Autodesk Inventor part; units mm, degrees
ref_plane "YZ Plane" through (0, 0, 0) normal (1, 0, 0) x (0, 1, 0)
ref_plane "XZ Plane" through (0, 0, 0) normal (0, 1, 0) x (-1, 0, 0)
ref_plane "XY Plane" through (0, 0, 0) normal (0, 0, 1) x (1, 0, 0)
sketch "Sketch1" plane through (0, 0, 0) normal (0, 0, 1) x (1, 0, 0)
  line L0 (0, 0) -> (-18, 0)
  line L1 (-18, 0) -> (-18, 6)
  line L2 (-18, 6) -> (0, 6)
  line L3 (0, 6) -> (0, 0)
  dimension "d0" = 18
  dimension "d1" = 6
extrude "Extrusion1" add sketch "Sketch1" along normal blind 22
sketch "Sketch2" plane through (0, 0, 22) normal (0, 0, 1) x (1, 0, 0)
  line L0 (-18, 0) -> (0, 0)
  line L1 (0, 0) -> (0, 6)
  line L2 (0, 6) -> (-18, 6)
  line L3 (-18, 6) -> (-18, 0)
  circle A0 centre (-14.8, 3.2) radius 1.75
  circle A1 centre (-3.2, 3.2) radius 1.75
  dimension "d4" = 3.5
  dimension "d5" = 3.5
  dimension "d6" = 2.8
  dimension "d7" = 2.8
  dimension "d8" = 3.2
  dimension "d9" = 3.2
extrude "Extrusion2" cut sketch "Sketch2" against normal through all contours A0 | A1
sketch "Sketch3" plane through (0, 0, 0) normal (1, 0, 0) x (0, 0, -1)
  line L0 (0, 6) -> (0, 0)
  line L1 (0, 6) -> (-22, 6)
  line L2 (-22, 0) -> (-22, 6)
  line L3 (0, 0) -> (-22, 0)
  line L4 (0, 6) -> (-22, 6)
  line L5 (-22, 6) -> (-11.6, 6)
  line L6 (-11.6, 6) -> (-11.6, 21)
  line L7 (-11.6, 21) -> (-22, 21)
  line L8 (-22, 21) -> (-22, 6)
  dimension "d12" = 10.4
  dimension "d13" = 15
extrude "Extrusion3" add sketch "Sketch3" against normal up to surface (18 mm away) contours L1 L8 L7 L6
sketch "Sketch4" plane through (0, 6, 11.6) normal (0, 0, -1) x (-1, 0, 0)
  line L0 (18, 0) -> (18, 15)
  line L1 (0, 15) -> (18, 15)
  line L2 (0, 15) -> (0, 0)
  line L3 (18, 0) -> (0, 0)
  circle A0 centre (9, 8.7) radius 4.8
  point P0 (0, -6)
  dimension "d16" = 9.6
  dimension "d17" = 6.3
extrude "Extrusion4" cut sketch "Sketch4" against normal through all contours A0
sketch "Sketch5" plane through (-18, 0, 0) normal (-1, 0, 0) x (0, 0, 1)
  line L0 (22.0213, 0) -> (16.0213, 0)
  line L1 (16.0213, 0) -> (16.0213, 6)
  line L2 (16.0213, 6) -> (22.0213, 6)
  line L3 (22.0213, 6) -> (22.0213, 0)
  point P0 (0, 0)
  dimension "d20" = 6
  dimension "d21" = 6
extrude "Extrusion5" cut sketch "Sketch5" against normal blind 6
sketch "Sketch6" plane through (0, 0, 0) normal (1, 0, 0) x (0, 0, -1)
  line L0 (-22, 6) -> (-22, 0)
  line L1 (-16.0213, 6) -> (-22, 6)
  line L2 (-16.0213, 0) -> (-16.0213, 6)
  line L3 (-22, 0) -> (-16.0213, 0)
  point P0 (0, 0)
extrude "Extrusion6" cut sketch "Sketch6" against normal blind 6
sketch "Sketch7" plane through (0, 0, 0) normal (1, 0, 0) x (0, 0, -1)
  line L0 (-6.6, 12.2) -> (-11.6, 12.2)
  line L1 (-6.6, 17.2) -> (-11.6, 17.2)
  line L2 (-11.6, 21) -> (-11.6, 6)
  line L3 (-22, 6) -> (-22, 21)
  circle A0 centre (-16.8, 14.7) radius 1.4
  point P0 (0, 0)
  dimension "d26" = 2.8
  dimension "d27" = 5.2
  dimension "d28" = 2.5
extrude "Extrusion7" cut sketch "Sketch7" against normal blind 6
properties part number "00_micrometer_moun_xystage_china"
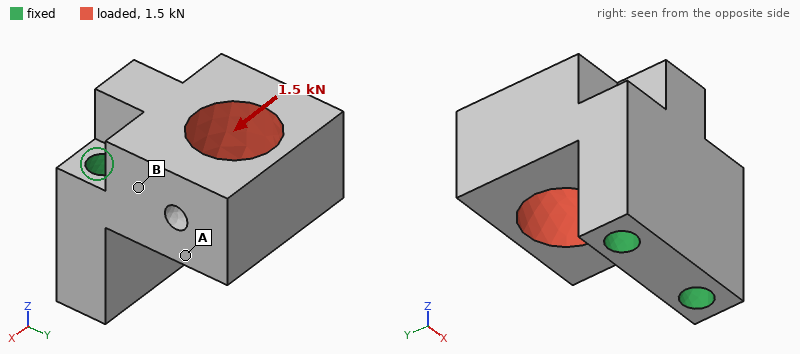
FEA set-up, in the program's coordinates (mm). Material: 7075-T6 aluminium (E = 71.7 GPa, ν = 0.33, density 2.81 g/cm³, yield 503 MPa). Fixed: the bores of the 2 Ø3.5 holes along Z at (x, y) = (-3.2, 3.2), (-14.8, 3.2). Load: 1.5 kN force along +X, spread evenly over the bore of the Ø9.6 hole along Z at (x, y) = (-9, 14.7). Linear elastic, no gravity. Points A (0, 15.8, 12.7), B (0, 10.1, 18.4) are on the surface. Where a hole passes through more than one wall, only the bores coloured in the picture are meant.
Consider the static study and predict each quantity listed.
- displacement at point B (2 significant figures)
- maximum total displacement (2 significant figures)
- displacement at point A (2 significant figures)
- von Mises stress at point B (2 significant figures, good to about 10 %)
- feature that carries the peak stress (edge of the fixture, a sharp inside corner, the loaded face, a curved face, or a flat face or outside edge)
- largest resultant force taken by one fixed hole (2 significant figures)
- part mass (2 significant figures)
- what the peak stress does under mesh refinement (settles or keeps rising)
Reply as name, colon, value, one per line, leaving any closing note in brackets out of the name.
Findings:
displacement at point B: 10 µm
maximum total displacement: 30 µm
displacement at point A: 20 µm
von Mises stress at point B: 26 MPa
feature that carries the peak stress: edge of the fixture
largest resultant force taken by one fixed hole: 1.5 kN
part mass: 10 g
what the peak stress does under mesh refinement: keeps rising
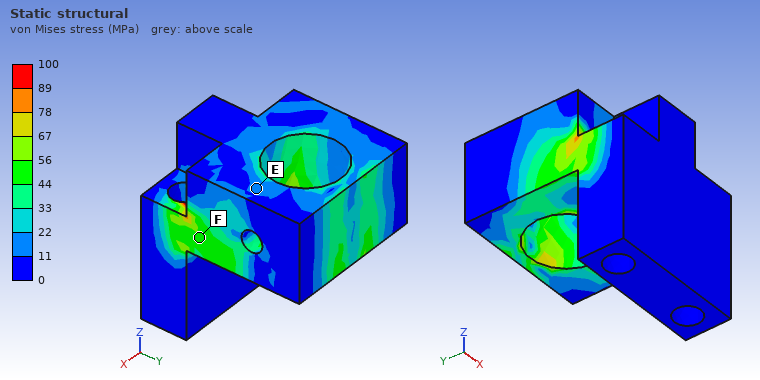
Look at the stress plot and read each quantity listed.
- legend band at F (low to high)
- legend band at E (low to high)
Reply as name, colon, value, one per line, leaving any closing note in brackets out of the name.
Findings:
legend band at F: 44 to 56 MPa
legend band at E: 11 to 22 MPa
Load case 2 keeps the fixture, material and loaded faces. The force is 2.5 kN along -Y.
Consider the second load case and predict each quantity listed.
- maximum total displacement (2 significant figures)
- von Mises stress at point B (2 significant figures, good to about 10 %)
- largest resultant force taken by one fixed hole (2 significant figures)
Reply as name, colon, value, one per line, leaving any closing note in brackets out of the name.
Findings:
maximum total displacement: 40 µm
von Mises stress at point B: 23 MPa
largest resultant force taken by one fixed hole: 1.3 kN
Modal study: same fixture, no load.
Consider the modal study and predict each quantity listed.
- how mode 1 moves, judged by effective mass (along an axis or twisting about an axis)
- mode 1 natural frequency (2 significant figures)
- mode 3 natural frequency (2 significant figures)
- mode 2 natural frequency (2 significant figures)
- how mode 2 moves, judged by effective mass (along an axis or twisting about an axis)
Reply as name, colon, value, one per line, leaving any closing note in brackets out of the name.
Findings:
how mode 1 moves, judged by effective mass: along Z
mode 1 natural frequency: 13 kHz
mode 3 natural frequency: 26 kHz
mode 2 natural frequency: 20 kHz
how mode 2 moves, judged by effective mass: along X
